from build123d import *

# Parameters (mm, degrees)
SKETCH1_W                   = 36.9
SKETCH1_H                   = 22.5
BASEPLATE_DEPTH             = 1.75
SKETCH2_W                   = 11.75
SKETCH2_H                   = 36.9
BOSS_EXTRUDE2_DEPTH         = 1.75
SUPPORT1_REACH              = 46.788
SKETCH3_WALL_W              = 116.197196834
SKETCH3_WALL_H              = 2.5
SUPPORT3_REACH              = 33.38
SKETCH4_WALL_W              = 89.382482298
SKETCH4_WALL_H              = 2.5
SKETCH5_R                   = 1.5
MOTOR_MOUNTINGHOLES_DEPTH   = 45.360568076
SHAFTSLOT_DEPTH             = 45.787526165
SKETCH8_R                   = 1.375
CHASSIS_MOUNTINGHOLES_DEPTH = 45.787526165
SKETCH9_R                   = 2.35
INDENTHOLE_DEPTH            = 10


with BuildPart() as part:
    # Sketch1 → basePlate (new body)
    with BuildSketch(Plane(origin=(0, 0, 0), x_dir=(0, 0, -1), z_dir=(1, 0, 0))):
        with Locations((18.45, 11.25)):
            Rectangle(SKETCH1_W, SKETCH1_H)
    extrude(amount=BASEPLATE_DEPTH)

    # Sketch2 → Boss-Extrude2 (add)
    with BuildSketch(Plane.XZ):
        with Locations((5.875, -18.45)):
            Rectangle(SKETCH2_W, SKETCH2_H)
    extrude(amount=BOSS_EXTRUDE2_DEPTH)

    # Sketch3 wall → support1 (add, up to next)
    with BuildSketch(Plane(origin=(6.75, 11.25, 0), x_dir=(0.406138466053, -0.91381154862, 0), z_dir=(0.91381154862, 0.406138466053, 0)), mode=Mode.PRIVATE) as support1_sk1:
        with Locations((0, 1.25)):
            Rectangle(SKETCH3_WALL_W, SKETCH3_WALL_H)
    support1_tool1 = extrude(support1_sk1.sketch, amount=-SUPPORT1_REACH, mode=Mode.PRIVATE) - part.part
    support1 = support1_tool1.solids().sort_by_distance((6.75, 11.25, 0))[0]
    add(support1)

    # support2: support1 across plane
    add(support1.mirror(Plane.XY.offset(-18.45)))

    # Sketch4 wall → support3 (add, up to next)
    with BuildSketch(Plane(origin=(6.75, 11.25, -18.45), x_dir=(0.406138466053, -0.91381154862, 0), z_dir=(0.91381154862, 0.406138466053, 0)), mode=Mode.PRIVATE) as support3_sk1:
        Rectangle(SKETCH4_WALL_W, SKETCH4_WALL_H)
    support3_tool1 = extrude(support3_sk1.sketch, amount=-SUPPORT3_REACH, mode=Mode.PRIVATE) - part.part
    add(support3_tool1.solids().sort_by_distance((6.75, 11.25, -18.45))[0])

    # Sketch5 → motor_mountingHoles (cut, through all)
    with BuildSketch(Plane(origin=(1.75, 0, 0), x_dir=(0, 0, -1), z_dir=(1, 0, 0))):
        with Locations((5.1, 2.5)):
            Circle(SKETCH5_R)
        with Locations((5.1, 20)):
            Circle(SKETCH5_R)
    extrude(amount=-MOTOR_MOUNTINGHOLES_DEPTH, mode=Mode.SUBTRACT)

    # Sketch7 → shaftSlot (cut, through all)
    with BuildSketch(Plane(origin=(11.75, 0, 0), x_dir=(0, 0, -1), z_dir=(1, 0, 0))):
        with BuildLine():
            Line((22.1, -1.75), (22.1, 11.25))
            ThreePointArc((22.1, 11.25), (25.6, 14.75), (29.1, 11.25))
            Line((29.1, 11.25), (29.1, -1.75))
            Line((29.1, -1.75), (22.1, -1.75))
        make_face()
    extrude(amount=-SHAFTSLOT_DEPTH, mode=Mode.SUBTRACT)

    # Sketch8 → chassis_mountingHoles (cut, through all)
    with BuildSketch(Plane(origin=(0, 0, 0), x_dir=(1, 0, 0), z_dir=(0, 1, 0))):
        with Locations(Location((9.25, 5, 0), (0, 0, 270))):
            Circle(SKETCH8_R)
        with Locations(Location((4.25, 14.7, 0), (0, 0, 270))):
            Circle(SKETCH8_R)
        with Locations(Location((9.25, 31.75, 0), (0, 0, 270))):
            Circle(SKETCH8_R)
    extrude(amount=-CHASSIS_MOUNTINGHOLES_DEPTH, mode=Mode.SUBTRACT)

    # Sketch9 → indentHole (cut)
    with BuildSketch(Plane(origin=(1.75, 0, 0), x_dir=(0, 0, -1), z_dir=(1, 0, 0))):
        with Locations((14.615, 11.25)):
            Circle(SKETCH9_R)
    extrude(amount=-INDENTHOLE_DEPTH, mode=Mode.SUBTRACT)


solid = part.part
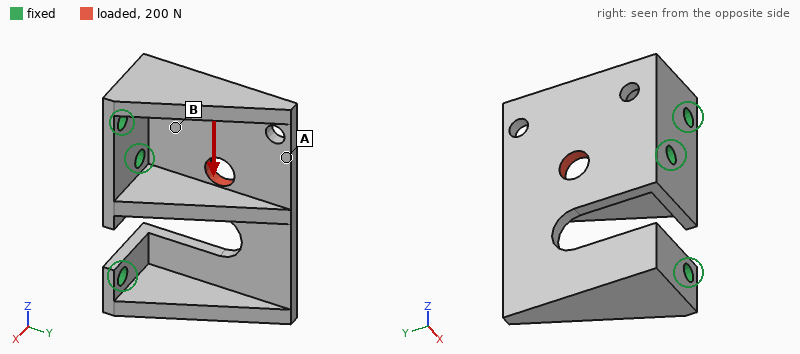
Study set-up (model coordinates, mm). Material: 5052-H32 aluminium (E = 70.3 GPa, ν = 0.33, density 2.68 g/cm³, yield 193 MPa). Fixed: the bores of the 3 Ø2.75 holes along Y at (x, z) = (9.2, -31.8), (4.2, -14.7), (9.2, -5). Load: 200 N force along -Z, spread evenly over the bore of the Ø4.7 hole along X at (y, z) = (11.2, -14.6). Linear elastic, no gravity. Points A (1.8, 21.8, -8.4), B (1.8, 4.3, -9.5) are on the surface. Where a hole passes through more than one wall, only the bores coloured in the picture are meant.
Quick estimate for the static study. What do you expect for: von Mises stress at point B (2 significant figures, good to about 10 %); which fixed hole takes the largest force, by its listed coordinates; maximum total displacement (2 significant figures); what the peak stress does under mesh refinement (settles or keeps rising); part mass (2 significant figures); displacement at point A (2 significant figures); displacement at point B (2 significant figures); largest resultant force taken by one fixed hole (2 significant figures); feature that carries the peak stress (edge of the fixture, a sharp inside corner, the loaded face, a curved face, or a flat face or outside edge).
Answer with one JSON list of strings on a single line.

["17 MPa", "(4.2, -14.7)", "46 µm", "keeps rising", "7.1 g", "34 µm", "10 µm", "150 N", "edge of the fixture"]
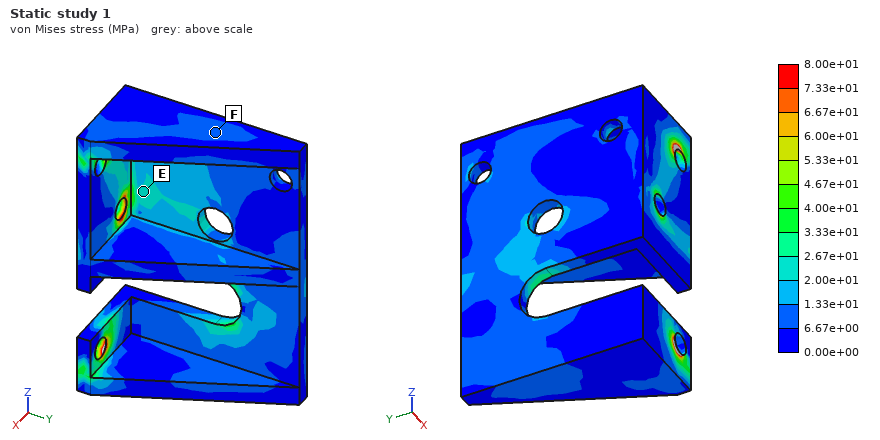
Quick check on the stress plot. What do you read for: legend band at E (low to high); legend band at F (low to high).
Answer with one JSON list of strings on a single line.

["2.00e+01 to 2.67e+01 MPa", "6.67e+00 to 1.33e+01 MPa"]
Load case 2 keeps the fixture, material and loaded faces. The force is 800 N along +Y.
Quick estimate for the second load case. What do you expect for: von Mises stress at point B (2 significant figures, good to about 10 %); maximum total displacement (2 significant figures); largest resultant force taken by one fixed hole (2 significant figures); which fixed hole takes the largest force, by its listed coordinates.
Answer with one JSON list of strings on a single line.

["28 MPa", "86 µm", "770 N", "(4.2, -14.7)"]
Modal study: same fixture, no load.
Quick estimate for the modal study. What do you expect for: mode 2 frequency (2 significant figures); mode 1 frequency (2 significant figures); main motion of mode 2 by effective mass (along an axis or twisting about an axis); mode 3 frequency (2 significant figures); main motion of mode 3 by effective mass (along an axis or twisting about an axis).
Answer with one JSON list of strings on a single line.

["5100 Hz", "4500 Hz", "along X", "11 kHz", "along Z"]
